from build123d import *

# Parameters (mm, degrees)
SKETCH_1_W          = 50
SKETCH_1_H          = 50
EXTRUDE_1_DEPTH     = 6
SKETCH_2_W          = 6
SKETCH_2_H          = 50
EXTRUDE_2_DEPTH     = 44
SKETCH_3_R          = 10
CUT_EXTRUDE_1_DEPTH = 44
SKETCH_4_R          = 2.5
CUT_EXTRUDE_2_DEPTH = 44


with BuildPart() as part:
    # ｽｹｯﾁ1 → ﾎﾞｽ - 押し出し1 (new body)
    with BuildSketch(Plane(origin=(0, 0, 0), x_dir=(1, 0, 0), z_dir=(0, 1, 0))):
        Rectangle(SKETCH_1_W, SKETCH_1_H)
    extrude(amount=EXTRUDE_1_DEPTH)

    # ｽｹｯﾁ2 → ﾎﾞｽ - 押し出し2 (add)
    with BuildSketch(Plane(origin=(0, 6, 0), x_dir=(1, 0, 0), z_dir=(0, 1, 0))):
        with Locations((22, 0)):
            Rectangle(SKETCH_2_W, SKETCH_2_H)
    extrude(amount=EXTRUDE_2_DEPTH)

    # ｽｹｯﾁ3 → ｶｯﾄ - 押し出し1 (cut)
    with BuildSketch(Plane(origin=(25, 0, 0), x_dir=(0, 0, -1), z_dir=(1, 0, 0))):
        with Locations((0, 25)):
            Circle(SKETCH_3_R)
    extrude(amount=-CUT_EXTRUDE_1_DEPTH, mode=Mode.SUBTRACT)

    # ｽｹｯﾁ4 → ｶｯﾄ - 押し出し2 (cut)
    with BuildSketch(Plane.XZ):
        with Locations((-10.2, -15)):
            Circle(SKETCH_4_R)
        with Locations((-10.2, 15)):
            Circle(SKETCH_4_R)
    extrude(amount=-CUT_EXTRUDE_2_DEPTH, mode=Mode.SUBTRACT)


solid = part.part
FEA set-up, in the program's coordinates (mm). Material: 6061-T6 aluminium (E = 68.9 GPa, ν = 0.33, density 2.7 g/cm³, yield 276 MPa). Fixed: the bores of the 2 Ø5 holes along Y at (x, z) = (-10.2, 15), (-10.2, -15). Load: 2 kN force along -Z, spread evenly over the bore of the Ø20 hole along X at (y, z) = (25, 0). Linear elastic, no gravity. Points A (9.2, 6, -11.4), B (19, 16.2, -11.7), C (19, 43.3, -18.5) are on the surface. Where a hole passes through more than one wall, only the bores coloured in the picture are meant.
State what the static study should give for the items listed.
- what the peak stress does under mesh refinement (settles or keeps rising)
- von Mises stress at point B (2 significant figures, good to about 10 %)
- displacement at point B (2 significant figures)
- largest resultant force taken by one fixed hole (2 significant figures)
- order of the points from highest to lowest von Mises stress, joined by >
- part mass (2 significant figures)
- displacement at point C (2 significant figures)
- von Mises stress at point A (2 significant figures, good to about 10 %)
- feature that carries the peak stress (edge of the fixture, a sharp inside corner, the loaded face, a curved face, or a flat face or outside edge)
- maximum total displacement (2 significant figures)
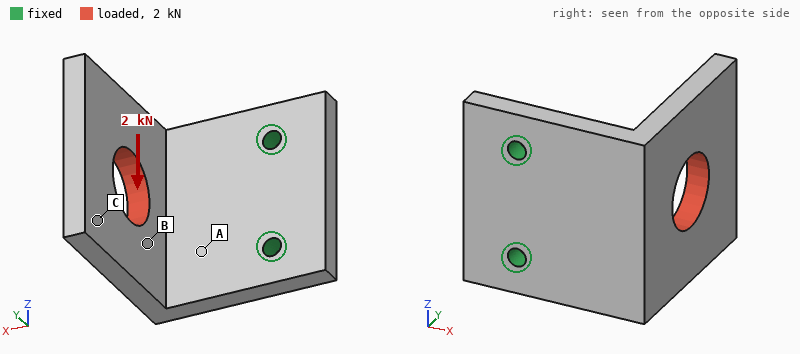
keeps rising
30 MPa
0.16 mm
2.5 kN
A > B > C
70 g
0.39 mm
95 MPa
edge of the fixture
0.46 mm
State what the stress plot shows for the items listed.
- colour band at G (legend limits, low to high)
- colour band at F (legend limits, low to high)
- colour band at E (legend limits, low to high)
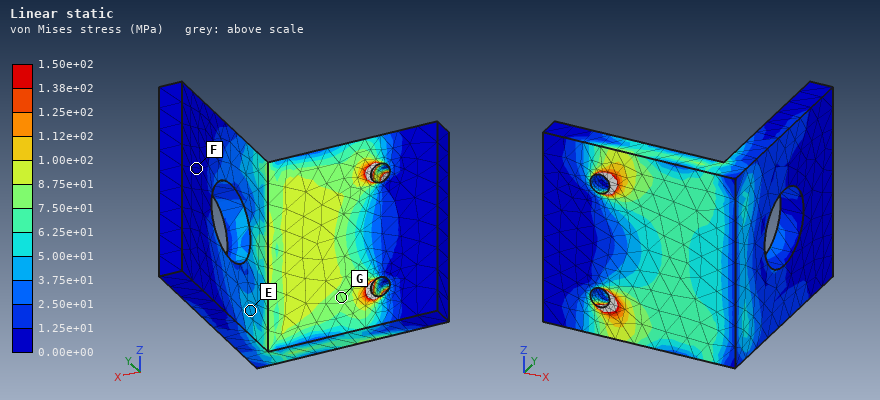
7.50e+01 to 8.75e+01 MPa
0.00e+00 to 1.25e+01 MPa
3.75e+01 to 5.00e+01 MPa
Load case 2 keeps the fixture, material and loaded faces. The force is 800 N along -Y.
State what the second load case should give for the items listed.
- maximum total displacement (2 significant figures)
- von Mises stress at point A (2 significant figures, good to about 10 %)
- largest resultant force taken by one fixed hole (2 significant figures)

0.35 mm
31 MPa
400 N
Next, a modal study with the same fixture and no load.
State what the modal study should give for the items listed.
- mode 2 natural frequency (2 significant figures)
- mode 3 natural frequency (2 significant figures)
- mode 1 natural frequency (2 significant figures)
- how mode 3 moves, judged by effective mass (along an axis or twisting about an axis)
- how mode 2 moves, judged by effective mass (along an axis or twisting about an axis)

1900 Hz
2900 Hz
1100 Hz
along Y
along Z
